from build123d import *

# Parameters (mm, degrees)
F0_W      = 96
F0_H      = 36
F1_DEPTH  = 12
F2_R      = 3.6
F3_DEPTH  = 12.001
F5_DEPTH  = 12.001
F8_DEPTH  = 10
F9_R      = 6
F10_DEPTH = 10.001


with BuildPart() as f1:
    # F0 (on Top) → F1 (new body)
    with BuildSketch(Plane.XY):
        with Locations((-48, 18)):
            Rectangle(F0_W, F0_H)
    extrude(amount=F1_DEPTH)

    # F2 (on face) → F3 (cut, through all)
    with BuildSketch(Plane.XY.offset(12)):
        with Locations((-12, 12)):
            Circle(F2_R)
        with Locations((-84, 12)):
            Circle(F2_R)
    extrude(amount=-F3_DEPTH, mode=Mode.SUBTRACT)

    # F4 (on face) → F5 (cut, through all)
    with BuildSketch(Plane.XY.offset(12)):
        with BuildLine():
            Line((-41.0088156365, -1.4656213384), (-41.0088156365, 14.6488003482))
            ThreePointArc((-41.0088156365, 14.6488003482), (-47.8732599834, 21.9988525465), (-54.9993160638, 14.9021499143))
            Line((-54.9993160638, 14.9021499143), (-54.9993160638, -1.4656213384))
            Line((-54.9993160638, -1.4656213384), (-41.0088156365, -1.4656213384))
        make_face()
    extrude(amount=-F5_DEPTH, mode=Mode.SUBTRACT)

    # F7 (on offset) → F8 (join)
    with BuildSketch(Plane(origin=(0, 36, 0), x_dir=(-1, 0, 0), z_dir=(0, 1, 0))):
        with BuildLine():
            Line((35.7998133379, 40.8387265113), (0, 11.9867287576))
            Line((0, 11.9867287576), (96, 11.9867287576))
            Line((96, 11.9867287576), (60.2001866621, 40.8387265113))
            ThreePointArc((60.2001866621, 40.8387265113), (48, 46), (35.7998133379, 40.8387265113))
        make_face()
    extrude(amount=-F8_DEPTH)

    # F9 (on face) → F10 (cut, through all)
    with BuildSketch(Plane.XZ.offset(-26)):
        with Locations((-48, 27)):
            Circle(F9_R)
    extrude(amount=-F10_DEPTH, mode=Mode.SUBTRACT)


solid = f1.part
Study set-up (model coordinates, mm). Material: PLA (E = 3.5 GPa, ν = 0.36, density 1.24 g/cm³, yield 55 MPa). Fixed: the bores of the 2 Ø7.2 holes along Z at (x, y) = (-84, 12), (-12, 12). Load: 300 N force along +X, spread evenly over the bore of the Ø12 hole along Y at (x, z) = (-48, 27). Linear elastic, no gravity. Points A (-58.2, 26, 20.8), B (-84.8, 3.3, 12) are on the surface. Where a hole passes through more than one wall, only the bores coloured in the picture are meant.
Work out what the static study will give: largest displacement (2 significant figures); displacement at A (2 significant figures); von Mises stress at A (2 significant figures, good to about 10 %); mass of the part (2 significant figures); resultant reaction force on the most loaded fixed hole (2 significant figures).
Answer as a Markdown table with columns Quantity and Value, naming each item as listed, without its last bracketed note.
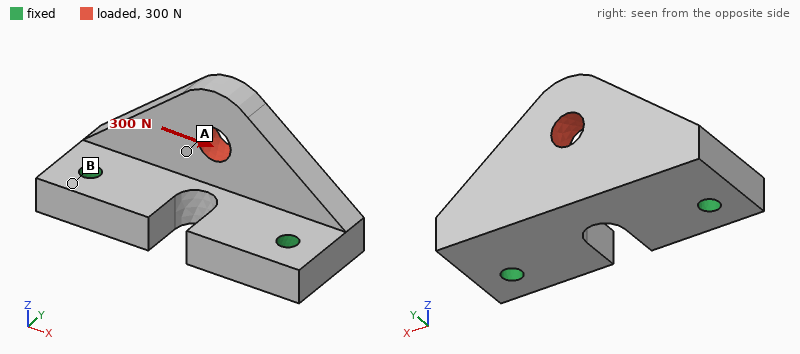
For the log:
| Quantity | Value |
|---|---|
| largest displacement | 30 µm |
| displacement at A | 17 µm |
| von Mises stress at A | 1.0 MPa |
| mass of the part | 67 g |
| resultant reaction force on the most loaded fixed hole | 180 N |
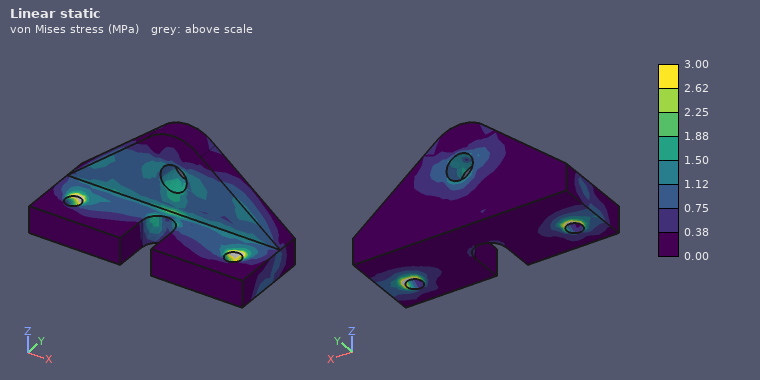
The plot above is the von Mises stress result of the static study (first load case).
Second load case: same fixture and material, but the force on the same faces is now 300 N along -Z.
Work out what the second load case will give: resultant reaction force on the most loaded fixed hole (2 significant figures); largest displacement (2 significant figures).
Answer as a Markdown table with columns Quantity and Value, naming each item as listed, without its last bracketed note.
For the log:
| Quantity | Value |
|---|---|
| resultant reaction force on the most loaded fixed hole | 150 N |
| largest displacement | 0.10 mm |
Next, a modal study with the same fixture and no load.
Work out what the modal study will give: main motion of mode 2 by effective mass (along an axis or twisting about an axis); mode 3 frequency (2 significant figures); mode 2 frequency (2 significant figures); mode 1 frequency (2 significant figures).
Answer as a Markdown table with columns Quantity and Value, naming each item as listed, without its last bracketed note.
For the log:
| Quantity | Value |
|---|---|
| main motion of mode 2 by effective mass | along Z |
| mode 3 frequency | 3100 Hz |
| mode 2 frequency | 3000 Hz |
| mode 1 frequency | 1500 Hz |
